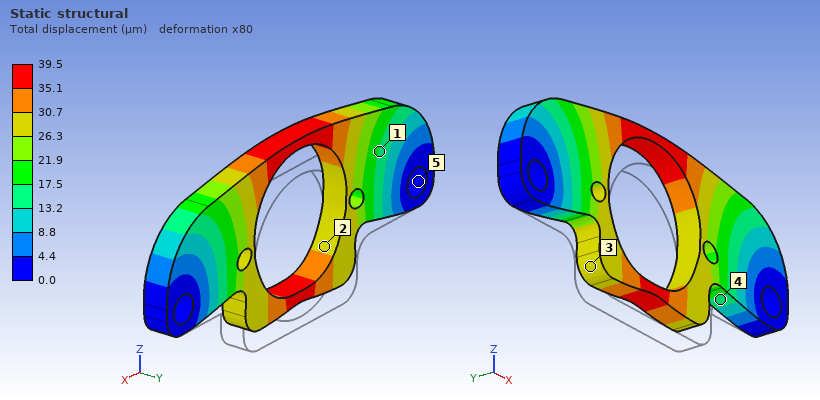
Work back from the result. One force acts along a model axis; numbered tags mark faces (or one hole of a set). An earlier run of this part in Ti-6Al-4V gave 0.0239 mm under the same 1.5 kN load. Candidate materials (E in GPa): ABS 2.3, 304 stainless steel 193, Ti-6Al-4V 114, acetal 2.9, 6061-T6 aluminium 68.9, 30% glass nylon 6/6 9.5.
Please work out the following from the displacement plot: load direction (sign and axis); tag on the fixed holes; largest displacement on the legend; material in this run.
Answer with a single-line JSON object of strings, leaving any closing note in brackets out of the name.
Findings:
{"load direction": "+Z", "tag on the fixed holes": "5", "largest displacement on the legend": "39.5 µm", "material in this run": "6061-T6 aluminium"}
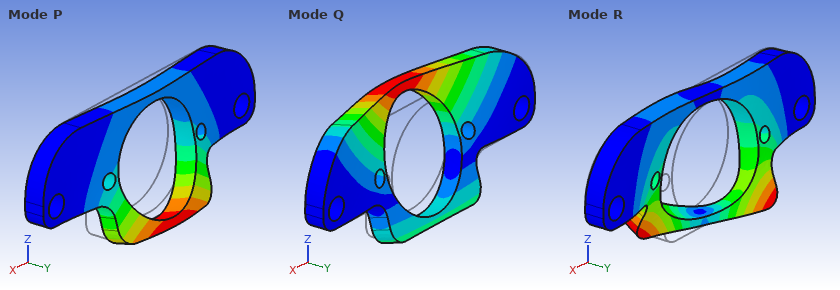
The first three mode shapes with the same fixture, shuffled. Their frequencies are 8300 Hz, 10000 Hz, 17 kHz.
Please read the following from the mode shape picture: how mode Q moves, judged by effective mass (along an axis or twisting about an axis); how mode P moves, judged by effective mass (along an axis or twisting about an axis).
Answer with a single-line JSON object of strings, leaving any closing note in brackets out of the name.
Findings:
{"how mode Q moves, judged by effective mass": "along Y", "how mode P moves, judged by effective mass": "along Y"}
